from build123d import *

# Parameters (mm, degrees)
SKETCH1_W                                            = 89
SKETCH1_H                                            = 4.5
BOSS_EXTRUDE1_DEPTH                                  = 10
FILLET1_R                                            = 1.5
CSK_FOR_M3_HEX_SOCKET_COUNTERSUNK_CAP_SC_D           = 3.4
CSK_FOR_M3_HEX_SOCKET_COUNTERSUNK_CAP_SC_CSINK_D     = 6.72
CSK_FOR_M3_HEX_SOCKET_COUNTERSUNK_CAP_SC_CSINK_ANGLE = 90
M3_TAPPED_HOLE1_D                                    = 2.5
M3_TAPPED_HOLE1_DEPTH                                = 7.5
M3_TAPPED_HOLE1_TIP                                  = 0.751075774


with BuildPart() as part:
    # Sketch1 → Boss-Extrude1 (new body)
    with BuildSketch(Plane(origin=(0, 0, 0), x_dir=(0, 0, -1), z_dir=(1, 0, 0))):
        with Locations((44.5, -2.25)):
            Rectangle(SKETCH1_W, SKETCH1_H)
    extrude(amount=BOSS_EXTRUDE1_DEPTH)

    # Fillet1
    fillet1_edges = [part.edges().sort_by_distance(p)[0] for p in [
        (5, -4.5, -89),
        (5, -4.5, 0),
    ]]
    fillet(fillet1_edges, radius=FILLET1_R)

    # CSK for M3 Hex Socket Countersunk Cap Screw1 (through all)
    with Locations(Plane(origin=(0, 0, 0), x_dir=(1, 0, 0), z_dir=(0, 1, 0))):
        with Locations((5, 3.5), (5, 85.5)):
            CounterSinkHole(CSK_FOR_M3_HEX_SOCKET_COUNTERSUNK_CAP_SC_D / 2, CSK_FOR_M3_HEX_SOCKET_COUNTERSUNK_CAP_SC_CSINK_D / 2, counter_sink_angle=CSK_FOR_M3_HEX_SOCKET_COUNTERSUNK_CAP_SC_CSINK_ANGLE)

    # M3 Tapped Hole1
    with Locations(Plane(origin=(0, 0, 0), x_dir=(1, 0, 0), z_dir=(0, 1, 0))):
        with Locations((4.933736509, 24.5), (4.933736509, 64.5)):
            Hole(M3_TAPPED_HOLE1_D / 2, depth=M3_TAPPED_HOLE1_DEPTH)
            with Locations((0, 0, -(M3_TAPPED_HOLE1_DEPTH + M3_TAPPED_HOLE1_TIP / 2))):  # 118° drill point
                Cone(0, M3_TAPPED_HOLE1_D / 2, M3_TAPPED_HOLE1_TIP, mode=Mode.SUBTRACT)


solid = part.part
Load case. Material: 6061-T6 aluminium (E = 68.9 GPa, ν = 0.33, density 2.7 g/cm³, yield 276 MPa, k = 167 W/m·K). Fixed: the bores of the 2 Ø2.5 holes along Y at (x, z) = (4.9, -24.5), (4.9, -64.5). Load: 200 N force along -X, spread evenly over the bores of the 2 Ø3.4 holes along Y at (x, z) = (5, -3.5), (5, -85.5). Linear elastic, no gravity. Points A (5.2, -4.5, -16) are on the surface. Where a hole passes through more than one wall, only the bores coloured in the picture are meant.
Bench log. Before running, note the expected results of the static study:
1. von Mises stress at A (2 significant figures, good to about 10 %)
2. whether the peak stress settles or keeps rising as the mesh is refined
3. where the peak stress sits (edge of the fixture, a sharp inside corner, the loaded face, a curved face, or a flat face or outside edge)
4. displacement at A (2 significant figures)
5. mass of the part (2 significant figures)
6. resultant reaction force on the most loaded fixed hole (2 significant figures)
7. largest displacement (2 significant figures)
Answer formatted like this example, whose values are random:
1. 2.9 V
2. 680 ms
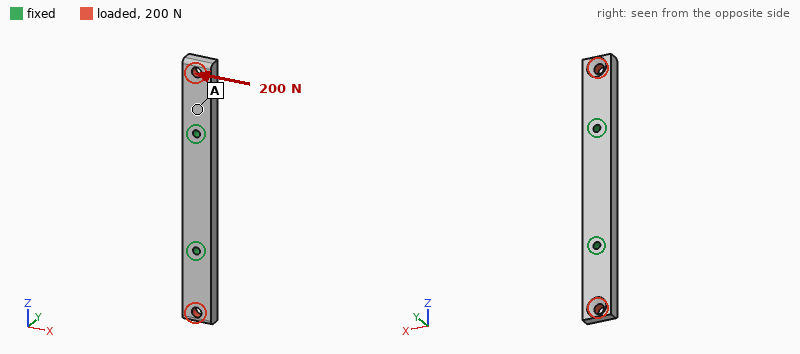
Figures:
1. 8.7 MPa
2. keeps rising
3. edge of the fixture
4. 7.8 µm
5. 10 g
6. 100 N
7. 31 µm
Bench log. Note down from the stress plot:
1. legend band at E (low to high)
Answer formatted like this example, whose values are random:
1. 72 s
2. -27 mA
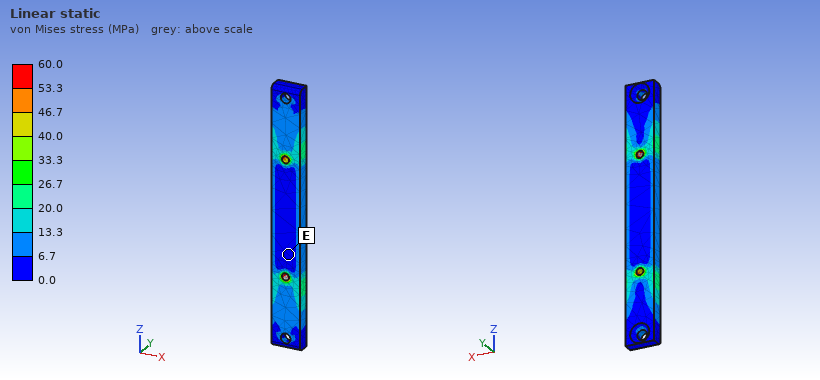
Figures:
1. 0.0 to 6.7 MPa
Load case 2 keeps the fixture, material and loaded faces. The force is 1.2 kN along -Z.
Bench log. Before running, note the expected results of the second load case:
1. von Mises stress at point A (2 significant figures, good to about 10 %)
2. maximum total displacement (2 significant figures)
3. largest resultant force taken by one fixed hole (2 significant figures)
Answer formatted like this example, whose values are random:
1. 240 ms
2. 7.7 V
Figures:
1. 29 MPa
2. 29 µm
3. 600 N
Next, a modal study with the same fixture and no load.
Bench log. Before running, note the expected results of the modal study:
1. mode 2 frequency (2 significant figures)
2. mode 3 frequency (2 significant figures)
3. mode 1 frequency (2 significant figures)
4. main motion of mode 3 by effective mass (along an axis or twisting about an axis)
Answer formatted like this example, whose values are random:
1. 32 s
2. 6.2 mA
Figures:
1. 6500 Hz
2. 9300 Hz
3. 6400 Hz
4. along X
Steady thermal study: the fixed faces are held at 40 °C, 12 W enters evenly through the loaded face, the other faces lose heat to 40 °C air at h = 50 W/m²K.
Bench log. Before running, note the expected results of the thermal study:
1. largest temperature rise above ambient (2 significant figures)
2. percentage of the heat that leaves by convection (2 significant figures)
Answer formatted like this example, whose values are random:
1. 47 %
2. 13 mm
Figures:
1. 19 K
2. 6.2 %
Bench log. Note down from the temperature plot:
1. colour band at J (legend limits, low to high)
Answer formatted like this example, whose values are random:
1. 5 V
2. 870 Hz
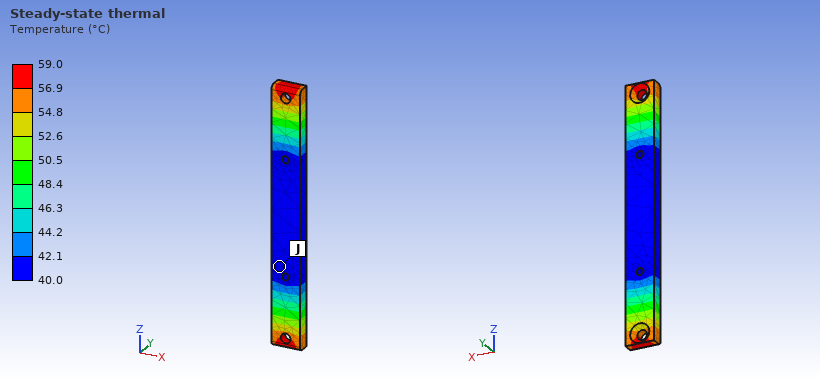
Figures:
1. 40.0 to 42.1 °C
